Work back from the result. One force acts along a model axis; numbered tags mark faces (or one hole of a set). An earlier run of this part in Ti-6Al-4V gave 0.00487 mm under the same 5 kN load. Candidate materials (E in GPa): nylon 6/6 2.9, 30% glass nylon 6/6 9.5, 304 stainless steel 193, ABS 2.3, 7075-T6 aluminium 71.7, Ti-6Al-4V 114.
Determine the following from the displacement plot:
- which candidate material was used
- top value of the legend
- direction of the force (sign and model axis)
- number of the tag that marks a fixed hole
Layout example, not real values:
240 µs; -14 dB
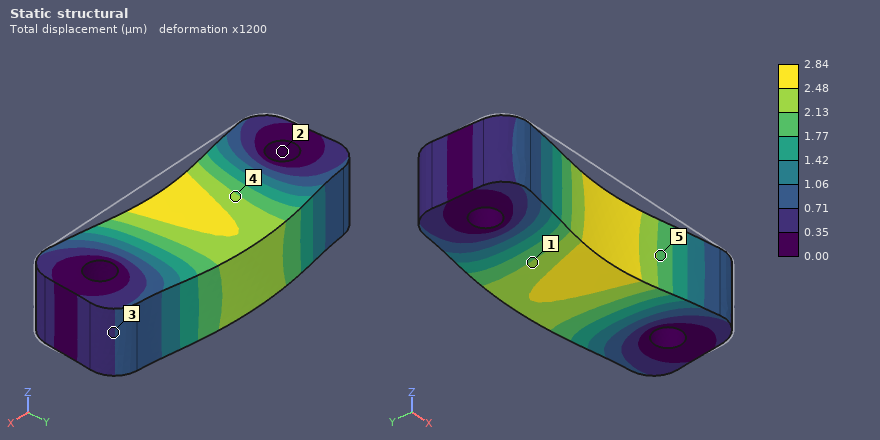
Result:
304 stainless steel; 2.84 µm; +Y; 2
